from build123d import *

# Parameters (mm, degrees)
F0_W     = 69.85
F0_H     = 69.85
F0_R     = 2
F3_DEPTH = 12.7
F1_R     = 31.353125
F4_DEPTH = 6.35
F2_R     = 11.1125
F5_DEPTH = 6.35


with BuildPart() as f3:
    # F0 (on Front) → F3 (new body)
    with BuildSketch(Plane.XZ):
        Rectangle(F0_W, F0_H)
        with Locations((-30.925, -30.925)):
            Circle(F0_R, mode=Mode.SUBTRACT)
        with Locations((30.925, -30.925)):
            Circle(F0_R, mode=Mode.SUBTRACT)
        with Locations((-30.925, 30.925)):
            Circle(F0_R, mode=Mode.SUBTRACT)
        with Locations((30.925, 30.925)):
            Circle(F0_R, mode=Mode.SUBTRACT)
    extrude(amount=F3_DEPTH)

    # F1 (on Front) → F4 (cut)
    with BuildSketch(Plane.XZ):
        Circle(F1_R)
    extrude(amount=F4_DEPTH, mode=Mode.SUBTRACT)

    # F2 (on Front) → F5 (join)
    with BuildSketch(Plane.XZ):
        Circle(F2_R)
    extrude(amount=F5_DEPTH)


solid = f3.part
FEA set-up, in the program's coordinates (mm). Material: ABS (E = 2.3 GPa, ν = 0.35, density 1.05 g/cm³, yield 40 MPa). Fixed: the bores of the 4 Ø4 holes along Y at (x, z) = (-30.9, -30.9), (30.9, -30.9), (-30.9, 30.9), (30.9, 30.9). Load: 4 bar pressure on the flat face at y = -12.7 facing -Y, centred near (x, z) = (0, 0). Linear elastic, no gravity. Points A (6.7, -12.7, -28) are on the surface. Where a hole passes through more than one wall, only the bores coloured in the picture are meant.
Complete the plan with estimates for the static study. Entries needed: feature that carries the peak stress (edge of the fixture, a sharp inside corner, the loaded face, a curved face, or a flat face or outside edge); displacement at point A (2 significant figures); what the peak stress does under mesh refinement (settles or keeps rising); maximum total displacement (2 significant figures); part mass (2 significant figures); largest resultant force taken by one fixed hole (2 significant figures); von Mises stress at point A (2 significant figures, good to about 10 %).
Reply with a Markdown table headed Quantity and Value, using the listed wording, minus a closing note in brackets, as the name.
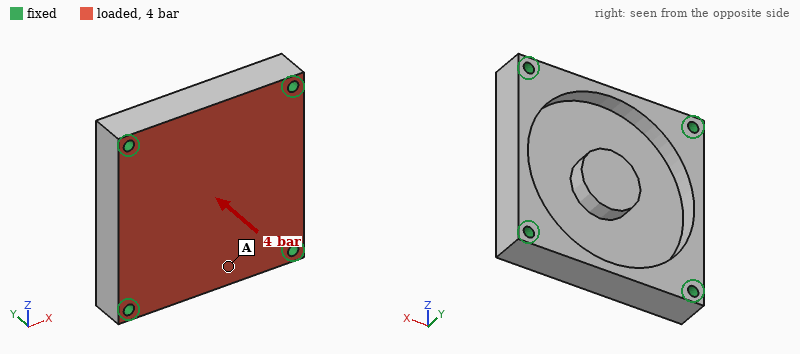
| Quantity | Value |
|---|---|
| feature that carries the peak stress | edge of the fixture |
| displacement at point A | 0.15 mm |
| what the peak stress does under mesh refinement | keeps rising |
| maximum total displacement | 0.31 mm |
| part mass | 46 g |
| largest resultant force taken by one fixed hole | 540 N |
| von Mises stress at point A | 4.9 MPa |
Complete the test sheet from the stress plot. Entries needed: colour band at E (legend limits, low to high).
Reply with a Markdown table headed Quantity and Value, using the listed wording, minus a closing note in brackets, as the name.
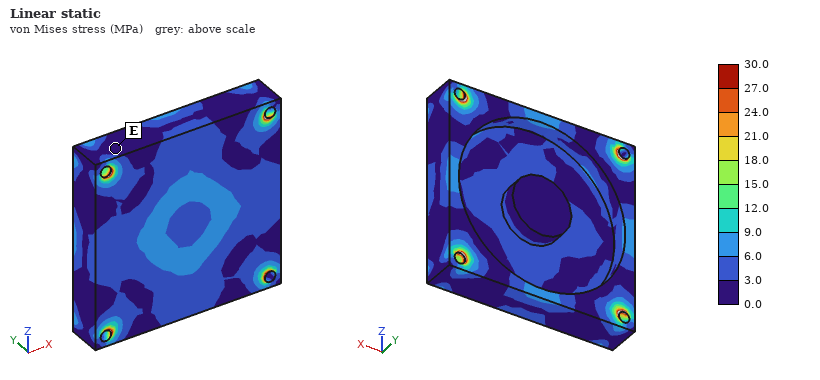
| Quantity | Value |
|---|---|
| colour band at E | 0.0 to 3.0 MPa |
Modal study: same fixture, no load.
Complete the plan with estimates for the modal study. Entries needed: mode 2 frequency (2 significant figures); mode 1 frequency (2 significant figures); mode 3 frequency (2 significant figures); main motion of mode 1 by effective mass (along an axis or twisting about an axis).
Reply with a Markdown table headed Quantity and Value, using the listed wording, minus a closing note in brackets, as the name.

| Quantity | Value |
|---|---|
| mode 2 frequency | 3800 Hz |
| mode 1 frequency | 2300 Hz |
| mode 3 frequency | 3800 Hz |
| main motion of mode 1 by effective mass | along Y |
